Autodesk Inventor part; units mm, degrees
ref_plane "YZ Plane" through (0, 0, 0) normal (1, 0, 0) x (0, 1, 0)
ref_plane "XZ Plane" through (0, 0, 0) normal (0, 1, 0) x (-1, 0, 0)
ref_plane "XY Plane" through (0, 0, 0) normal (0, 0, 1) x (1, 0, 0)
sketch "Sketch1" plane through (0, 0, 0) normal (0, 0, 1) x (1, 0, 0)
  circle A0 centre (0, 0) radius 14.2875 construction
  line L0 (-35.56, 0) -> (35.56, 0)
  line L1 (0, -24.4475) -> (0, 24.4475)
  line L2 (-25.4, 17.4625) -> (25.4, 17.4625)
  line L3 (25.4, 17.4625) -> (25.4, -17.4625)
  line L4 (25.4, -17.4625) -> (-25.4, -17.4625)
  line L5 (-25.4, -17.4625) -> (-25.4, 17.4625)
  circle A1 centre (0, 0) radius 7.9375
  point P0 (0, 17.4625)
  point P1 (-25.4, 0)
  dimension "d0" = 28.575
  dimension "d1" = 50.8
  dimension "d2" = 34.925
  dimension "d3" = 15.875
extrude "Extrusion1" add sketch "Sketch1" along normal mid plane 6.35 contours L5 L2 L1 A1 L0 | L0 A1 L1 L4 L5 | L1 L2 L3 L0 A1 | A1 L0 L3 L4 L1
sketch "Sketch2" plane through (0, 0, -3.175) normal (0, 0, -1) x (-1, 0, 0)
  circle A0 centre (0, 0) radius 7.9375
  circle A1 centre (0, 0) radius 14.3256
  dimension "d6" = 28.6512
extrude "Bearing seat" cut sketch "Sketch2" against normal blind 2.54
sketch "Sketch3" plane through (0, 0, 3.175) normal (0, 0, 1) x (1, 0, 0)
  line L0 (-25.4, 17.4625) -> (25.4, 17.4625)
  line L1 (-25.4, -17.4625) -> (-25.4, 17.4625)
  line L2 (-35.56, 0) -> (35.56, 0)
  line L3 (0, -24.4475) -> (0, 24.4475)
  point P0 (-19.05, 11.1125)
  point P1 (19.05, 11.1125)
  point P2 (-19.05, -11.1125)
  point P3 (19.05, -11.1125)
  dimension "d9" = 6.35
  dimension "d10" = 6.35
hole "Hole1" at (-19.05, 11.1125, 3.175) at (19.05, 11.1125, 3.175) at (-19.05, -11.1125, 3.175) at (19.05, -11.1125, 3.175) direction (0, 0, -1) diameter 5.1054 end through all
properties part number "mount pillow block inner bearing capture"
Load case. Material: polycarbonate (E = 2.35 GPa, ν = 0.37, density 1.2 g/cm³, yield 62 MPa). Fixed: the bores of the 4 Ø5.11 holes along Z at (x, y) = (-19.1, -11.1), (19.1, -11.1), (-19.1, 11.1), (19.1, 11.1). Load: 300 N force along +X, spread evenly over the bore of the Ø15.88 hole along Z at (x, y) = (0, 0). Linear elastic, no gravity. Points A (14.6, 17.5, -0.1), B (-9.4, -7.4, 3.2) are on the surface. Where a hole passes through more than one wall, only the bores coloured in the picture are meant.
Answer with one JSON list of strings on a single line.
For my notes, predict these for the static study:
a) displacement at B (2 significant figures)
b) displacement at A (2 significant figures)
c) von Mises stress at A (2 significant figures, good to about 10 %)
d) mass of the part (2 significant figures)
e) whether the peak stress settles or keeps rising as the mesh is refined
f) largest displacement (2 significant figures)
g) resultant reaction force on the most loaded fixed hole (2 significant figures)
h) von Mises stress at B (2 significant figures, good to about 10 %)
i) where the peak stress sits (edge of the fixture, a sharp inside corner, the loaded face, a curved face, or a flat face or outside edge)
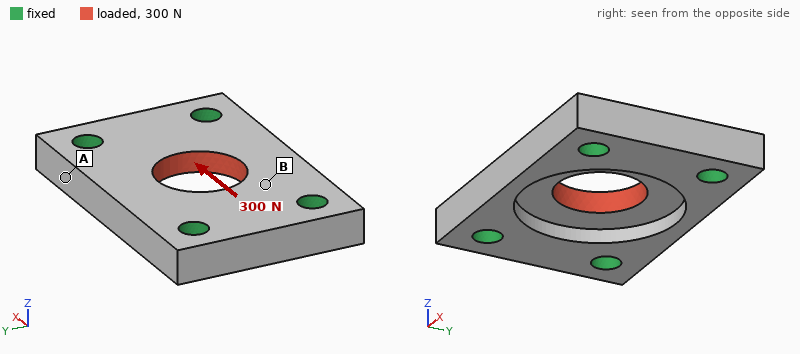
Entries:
["6.4 µm", "2.1 µm", "0.37 MPa", "10 g", "keeps rising", "11 µm", "78 N", "1.4 MPa", "edge of the fixture"]
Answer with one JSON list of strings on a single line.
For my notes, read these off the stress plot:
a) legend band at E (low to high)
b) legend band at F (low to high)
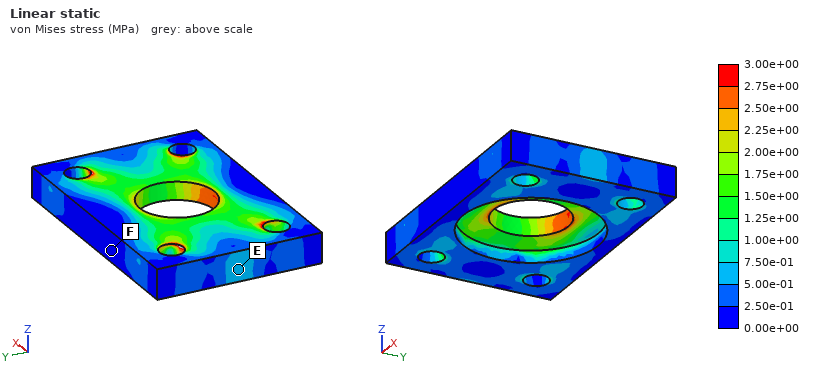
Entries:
["5.00e-01 to 7.50e-01 MPa", "0.00e+00 to 2.50e-01 MPa"]
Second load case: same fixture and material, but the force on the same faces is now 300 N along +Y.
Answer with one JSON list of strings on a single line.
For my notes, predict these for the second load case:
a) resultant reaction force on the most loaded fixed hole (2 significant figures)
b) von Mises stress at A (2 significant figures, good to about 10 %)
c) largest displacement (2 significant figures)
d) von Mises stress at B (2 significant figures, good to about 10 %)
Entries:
["84 N", "1.0 MPa", "26 µm", "1.8 MPa"]
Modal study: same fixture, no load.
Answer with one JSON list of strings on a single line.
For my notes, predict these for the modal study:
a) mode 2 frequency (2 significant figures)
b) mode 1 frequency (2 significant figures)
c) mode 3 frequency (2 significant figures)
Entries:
["6700 Hz", "6400 Hz", "9800 Hz"]
